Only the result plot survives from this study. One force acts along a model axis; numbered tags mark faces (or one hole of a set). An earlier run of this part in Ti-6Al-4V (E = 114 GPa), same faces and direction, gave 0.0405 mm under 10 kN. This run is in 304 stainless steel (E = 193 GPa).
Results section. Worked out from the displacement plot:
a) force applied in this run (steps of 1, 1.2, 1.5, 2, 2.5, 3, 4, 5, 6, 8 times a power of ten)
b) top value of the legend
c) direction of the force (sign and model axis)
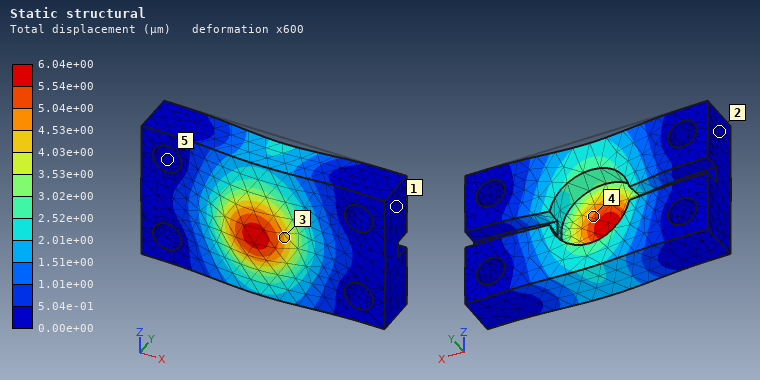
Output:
2.5 kN
6.04e+00 µm
-Y
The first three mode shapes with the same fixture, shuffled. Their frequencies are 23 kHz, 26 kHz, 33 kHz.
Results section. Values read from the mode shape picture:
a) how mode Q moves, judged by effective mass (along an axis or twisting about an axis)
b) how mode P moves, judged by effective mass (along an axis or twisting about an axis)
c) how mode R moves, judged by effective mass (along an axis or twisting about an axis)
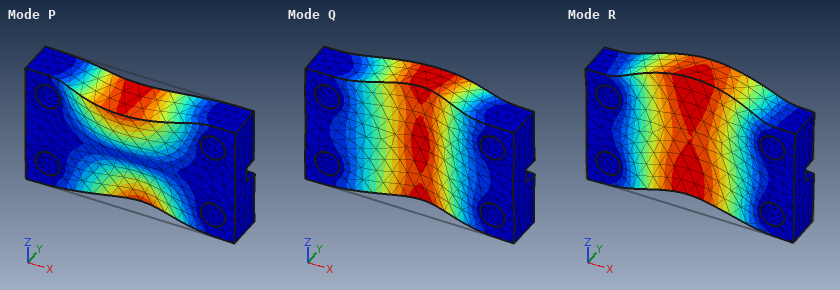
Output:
along Y
twisting about X
along Z
